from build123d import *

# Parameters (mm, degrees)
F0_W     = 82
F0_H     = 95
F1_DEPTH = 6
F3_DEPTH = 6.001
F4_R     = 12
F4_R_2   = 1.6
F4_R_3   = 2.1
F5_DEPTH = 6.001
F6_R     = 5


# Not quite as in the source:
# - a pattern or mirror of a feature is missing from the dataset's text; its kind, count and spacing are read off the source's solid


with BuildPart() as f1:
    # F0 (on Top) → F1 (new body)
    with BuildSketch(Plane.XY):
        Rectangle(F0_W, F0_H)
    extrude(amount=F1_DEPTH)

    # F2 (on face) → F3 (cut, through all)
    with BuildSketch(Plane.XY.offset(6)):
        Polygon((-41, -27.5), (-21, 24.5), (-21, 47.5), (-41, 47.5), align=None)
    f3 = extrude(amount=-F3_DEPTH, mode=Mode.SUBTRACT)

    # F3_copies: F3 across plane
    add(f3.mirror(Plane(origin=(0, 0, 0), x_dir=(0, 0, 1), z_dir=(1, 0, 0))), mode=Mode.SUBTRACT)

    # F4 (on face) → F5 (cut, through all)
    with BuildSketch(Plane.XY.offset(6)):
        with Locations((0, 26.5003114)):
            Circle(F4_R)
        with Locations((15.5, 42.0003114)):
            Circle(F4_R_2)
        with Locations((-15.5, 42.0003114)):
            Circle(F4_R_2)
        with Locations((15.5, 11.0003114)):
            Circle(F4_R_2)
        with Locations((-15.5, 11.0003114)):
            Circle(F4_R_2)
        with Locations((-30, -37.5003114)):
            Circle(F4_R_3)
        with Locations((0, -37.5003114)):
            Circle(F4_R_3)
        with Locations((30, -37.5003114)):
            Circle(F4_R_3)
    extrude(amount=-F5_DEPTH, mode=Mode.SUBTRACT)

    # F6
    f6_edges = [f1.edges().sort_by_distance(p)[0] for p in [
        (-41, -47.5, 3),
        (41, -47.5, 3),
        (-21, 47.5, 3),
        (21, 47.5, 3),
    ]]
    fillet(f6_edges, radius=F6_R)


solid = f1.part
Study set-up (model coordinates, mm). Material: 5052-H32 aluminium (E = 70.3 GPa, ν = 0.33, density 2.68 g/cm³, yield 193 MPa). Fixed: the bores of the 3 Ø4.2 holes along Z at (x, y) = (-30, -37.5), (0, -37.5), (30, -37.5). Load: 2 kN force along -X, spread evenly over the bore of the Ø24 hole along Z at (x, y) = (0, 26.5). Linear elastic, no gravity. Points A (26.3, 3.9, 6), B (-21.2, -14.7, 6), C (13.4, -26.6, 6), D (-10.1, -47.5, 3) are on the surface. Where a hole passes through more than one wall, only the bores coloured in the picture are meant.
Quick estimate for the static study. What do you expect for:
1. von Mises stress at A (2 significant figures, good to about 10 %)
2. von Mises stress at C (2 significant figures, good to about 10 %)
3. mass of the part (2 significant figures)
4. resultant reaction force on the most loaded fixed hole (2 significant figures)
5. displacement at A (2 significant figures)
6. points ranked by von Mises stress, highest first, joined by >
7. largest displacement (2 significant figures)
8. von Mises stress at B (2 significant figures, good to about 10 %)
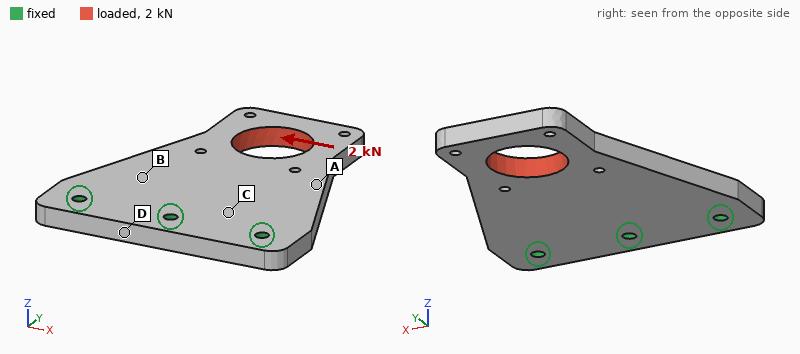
18 MPa
8.8 MPa
85 g
2.2 kN
17 µm
A > B > C > D
56 µm
12 MPa
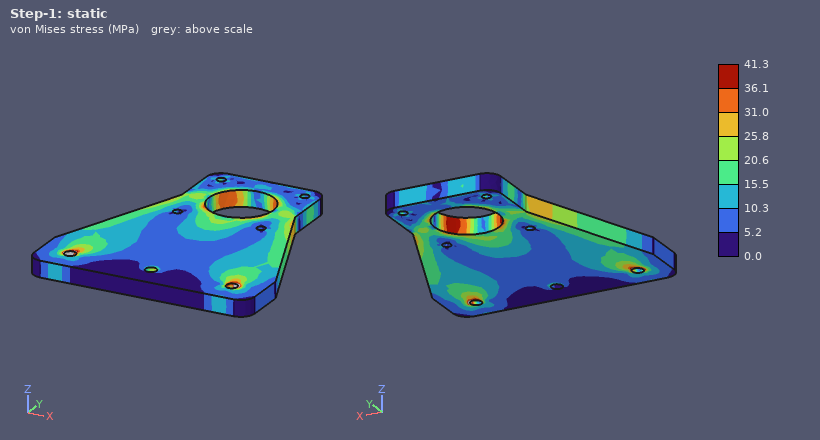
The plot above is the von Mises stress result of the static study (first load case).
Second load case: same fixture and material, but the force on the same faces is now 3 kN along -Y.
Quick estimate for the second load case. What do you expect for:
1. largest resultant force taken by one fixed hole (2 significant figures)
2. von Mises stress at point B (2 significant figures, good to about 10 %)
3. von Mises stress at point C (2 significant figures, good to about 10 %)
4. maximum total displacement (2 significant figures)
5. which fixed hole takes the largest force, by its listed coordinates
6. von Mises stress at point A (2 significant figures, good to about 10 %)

1.1 kN
7.2 MPa
4.7 MPa
17 µm
(0, -37.5)
10 MPa
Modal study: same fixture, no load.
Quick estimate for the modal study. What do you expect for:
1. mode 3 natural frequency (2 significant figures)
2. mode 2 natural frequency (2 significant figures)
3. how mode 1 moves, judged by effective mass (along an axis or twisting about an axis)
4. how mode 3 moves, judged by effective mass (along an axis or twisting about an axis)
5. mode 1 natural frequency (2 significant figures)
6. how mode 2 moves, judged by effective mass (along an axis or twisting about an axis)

3900 Hz
3100 Hz
along Z
along Z
960 Hz
twisting about Y
